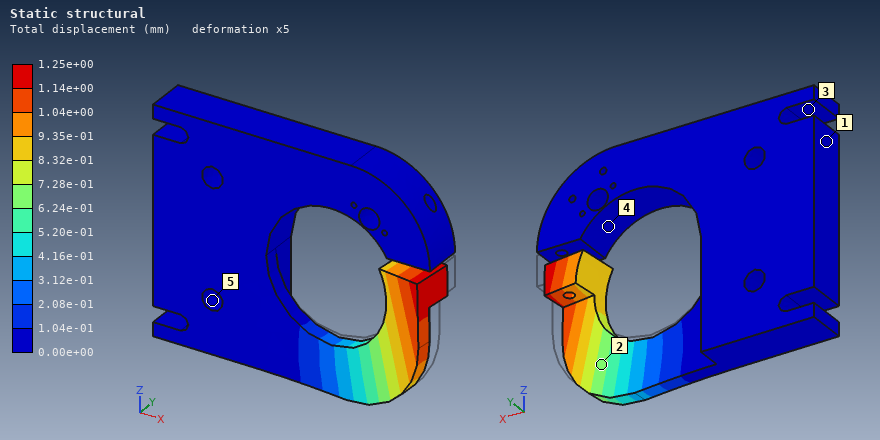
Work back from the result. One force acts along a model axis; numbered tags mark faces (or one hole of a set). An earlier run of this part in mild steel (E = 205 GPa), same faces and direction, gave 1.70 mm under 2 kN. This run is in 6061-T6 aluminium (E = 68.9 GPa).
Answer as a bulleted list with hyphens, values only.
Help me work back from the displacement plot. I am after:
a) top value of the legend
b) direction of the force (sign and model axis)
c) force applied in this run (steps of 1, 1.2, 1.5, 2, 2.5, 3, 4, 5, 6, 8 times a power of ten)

- 1.25e+00 mm
- -Y
- 500 N
